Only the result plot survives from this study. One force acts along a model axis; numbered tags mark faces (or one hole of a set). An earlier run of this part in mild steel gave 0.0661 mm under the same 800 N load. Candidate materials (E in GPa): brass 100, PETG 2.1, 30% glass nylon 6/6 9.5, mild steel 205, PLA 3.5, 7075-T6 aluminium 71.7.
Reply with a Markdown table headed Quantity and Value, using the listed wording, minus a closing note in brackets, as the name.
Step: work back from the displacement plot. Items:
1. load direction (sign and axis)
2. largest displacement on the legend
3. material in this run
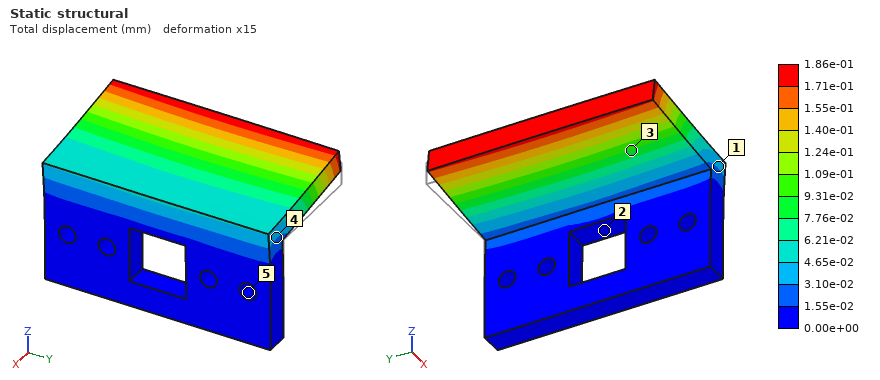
| Quantity | Value |
|---|---|
| load direction | +Z |
| largest displacement on the legend | 1.86e-01 mm |
| material in this run | 7075-T6 aluminium |
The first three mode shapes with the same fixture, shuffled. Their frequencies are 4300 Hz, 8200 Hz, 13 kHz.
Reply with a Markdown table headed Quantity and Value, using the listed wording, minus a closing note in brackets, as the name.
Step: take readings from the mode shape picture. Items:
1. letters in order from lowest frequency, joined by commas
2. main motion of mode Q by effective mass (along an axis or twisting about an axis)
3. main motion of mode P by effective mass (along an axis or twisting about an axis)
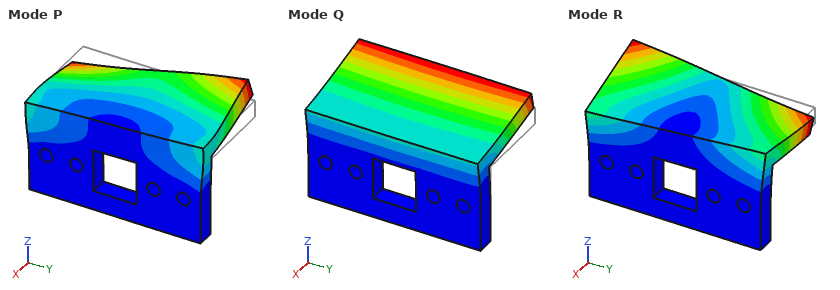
| Quantity | Value |
|---|---|
| letters in order from lowest frequency, joined by commas | Q, R, P |
| main motion of mode Q by effective mass | along Z |
| main motion of mode P by effective mass | along Y |
